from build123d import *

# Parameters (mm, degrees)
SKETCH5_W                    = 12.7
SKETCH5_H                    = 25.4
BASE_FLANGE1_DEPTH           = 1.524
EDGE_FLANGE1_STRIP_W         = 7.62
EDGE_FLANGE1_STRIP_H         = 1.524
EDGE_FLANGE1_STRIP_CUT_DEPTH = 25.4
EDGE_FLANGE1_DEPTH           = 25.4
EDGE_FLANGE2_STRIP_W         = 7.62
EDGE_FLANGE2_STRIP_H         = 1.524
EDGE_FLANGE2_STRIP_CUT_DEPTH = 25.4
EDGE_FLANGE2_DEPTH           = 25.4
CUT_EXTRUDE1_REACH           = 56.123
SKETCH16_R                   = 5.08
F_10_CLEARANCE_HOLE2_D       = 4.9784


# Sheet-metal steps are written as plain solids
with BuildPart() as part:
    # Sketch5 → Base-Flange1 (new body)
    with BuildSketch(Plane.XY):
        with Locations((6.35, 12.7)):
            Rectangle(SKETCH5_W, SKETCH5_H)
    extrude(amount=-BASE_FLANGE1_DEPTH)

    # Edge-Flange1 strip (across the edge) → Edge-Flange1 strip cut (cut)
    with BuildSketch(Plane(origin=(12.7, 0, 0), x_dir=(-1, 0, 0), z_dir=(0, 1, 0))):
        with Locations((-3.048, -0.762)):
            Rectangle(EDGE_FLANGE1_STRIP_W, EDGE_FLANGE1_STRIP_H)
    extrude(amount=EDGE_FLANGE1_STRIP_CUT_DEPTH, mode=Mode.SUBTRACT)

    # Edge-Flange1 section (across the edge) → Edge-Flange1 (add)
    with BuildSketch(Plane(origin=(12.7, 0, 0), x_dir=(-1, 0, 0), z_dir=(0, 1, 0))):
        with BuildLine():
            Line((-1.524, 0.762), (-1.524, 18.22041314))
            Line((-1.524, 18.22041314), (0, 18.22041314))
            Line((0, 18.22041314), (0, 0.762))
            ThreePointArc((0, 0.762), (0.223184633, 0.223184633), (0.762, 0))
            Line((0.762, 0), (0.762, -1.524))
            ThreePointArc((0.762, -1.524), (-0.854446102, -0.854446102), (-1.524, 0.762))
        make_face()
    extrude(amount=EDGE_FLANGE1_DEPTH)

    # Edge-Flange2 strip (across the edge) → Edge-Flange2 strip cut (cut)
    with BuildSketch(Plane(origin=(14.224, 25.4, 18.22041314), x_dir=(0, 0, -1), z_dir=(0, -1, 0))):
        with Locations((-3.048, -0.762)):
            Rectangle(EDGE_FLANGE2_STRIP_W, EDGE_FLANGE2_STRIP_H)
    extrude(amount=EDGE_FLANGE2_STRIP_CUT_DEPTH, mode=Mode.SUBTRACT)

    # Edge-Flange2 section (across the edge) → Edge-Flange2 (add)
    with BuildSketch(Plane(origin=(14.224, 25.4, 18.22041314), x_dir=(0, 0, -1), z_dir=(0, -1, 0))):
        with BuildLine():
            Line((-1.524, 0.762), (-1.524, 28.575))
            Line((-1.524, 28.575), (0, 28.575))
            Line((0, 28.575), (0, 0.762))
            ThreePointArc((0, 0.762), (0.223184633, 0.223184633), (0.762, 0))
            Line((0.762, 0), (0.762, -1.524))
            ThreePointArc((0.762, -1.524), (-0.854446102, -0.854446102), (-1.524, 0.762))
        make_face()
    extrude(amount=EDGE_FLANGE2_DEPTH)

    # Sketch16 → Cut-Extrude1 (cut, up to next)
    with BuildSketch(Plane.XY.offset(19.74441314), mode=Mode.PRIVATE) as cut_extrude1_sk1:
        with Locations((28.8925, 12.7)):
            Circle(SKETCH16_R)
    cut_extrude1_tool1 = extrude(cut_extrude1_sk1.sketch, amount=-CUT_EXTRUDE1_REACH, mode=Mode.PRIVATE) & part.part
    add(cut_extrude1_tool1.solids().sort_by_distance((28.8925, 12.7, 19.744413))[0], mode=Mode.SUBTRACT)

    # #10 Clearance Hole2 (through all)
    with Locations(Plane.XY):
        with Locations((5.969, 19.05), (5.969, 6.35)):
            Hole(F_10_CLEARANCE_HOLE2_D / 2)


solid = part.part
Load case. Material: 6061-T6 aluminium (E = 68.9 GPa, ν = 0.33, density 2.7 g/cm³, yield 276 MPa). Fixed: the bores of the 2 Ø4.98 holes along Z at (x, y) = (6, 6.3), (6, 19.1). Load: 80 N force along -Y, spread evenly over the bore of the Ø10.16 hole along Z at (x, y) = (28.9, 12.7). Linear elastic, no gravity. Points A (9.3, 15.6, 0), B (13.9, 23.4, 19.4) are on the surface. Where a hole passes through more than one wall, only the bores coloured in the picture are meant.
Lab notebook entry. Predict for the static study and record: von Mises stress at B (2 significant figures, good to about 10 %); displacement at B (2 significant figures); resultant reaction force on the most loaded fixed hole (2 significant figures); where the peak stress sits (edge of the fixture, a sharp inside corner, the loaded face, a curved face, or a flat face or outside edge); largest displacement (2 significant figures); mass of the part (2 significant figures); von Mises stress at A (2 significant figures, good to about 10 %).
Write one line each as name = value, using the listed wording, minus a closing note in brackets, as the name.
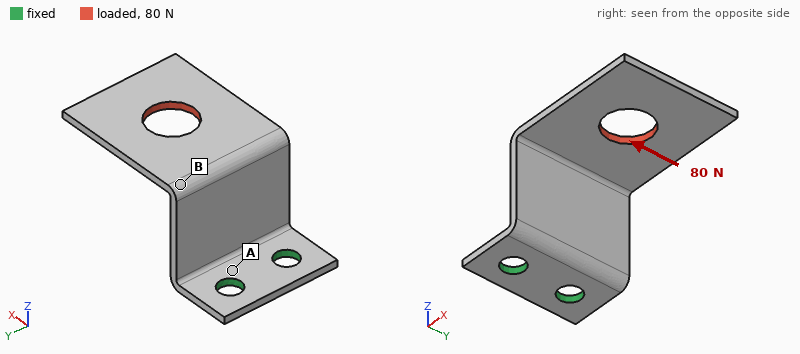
von Mises stress at B = 59 MPa
displacement at B = 0.21 mm
resultant reaction force on the most loaded fixed hole = 150 N
where the peak stress sits = a curved face
largest displacement = 0.63 mm
mass of the part = 5.9 g
von Mises stress at A = 13 MPa
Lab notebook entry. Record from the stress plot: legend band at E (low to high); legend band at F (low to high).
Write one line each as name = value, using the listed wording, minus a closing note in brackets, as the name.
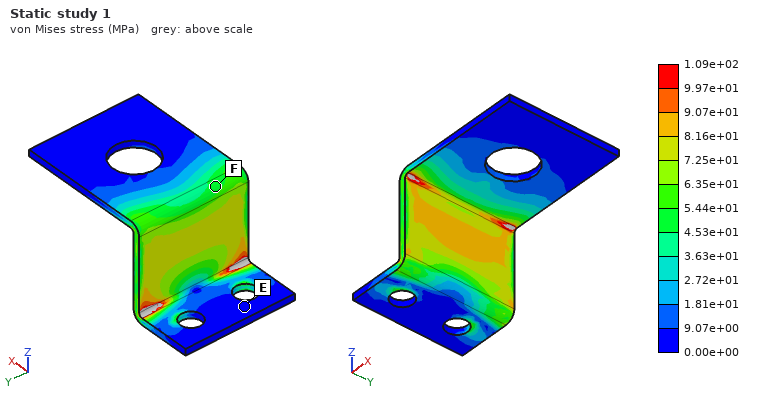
legend band at E = 0.00e+00 to 9.07e+00 MPa
legend band at F = 4.53e+01 to 5.44e+01 MPa
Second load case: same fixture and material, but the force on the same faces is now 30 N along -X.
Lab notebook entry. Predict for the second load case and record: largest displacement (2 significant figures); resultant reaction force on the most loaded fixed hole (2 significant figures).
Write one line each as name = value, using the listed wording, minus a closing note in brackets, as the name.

largest displacement = 0.55 mm
resultant reaction force on the most loaded fixed hole = 16 N
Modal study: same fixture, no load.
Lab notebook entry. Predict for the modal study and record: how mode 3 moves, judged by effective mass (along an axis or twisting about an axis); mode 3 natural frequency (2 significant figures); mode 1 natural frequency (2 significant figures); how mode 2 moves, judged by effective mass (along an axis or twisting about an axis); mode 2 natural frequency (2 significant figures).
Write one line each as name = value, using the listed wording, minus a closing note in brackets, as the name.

how mode 3 moves, judged by effective mass = along X
mode 3 natural frequency = 1800 Hz
mode 1 natural frequency = 610 Hz
how mode 2 moves, judged by effective mass = along Y
mode 2 natural frequency = 1300 Hz
